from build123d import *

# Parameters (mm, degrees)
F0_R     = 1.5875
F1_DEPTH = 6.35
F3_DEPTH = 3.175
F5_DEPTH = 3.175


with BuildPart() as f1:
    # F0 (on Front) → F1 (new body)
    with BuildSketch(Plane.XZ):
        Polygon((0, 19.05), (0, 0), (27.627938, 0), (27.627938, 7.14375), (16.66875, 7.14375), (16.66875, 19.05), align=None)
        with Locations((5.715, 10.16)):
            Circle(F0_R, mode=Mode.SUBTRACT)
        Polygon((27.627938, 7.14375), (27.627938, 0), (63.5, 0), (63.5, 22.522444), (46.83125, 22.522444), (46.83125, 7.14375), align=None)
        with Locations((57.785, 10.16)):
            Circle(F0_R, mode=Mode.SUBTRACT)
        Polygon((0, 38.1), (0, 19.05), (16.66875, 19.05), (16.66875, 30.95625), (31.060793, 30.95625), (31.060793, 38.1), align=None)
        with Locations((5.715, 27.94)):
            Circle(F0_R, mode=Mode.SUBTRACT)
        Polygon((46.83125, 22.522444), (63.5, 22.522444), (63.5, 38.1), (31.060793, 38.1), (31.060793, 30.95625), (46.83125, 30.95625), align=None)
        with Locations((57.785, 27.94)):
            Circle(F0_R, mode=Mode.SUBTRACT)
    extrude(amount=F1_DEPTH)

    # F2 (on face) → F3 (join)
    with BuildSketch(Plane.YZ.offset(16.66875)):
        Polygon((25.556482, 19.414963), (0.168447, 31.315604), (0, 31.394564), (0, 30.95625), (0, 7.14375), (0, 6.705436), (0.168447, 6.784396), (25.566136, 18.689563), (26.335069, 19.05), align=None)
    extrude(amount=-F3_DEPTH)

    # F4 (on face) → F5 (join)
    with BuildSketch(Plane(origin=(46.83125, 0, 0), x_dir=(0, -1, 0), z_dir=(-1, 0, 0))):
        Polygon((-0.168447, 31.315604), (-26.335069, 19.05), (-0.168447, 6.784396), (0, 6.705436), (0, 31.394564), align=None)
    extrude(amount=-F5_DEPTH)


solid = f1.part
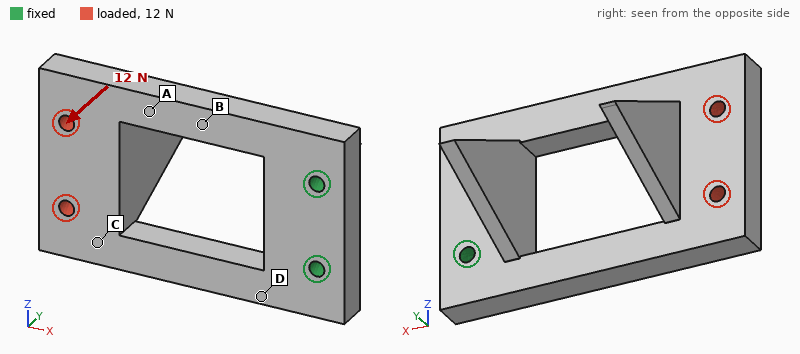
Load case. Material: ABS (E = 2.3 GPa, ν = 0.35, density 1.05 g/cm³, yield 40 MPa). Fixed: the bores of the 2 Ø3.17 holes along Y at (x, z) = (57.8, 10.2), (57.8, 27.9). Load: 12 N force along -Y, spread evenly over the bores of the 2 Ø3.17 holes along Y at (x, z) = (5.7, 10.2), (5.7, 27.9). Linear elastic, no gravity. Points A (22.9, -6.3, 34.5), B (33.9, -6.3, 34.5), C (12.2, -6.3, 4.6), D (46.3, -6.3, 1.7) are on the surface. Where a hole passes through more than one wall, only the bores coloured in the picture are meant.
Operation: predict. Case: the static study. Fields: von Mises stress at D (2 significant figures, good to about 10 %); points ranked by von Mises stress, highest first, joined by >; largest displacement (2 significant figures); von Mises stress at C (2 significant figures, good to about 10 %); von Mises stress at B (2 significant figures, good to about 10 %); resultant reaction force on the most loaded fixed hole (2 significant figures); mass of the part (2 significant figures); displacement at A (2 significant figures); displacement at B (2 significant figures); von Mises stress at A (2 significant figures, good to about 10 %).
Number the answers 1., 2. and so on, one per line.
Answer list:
1. 4.5 MPa
2. D > B > A > C
3. 0.80 mm
4. 0.66 MPa
5. 3.5 MPa
6. 6.2 N
7. 13 g
8. 0.34 mm
9. 0.17 mm
10. 2.2 MPa
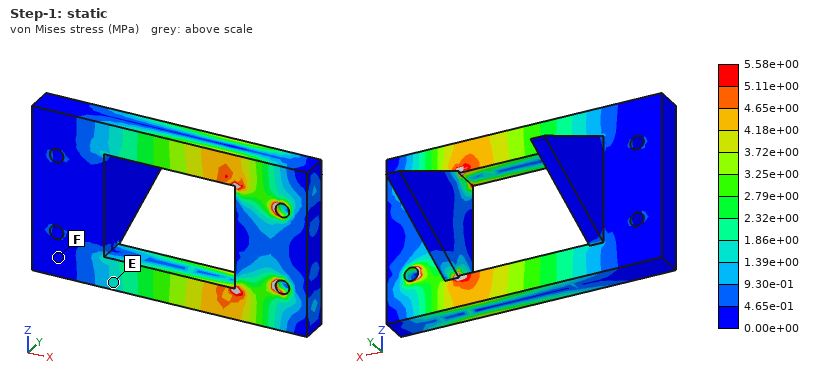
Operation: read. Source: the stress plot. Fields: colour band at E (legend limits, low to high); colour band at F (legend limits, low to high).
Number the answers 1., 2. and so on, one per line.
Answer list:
1. 1.39e+00 to 1.86e+00 MPa
2. 0.00e+00 to 4.65e-01 MPa
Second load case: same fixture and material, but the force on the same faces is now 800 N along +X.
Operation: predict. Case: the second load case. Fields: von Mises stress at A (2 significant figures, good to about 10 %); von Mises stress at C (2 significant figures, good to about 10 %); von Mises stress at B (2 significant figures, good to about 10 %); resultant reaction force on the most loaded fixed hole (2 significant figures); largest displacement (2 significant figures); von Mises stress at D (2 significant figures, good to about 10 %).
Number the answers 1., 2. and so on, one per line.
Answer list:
1. 8.8 MPa
2. 8.2 MPa
3. 8.8 MPa
4. 420 N
5. 0.34 mm
6. 7.7 MPa
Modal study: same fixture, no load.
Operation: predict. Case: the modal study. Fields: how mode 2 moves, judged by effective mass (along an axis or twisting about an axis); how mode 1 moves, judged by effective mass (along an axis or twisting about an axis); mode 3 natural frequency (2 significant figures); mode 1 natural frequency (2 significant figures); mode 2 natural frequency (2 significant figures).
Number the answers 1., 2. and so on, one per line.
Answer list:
1. along Z
2. along Y
3. 900 Hz
4. 310 Hz
5. 730 Hz
